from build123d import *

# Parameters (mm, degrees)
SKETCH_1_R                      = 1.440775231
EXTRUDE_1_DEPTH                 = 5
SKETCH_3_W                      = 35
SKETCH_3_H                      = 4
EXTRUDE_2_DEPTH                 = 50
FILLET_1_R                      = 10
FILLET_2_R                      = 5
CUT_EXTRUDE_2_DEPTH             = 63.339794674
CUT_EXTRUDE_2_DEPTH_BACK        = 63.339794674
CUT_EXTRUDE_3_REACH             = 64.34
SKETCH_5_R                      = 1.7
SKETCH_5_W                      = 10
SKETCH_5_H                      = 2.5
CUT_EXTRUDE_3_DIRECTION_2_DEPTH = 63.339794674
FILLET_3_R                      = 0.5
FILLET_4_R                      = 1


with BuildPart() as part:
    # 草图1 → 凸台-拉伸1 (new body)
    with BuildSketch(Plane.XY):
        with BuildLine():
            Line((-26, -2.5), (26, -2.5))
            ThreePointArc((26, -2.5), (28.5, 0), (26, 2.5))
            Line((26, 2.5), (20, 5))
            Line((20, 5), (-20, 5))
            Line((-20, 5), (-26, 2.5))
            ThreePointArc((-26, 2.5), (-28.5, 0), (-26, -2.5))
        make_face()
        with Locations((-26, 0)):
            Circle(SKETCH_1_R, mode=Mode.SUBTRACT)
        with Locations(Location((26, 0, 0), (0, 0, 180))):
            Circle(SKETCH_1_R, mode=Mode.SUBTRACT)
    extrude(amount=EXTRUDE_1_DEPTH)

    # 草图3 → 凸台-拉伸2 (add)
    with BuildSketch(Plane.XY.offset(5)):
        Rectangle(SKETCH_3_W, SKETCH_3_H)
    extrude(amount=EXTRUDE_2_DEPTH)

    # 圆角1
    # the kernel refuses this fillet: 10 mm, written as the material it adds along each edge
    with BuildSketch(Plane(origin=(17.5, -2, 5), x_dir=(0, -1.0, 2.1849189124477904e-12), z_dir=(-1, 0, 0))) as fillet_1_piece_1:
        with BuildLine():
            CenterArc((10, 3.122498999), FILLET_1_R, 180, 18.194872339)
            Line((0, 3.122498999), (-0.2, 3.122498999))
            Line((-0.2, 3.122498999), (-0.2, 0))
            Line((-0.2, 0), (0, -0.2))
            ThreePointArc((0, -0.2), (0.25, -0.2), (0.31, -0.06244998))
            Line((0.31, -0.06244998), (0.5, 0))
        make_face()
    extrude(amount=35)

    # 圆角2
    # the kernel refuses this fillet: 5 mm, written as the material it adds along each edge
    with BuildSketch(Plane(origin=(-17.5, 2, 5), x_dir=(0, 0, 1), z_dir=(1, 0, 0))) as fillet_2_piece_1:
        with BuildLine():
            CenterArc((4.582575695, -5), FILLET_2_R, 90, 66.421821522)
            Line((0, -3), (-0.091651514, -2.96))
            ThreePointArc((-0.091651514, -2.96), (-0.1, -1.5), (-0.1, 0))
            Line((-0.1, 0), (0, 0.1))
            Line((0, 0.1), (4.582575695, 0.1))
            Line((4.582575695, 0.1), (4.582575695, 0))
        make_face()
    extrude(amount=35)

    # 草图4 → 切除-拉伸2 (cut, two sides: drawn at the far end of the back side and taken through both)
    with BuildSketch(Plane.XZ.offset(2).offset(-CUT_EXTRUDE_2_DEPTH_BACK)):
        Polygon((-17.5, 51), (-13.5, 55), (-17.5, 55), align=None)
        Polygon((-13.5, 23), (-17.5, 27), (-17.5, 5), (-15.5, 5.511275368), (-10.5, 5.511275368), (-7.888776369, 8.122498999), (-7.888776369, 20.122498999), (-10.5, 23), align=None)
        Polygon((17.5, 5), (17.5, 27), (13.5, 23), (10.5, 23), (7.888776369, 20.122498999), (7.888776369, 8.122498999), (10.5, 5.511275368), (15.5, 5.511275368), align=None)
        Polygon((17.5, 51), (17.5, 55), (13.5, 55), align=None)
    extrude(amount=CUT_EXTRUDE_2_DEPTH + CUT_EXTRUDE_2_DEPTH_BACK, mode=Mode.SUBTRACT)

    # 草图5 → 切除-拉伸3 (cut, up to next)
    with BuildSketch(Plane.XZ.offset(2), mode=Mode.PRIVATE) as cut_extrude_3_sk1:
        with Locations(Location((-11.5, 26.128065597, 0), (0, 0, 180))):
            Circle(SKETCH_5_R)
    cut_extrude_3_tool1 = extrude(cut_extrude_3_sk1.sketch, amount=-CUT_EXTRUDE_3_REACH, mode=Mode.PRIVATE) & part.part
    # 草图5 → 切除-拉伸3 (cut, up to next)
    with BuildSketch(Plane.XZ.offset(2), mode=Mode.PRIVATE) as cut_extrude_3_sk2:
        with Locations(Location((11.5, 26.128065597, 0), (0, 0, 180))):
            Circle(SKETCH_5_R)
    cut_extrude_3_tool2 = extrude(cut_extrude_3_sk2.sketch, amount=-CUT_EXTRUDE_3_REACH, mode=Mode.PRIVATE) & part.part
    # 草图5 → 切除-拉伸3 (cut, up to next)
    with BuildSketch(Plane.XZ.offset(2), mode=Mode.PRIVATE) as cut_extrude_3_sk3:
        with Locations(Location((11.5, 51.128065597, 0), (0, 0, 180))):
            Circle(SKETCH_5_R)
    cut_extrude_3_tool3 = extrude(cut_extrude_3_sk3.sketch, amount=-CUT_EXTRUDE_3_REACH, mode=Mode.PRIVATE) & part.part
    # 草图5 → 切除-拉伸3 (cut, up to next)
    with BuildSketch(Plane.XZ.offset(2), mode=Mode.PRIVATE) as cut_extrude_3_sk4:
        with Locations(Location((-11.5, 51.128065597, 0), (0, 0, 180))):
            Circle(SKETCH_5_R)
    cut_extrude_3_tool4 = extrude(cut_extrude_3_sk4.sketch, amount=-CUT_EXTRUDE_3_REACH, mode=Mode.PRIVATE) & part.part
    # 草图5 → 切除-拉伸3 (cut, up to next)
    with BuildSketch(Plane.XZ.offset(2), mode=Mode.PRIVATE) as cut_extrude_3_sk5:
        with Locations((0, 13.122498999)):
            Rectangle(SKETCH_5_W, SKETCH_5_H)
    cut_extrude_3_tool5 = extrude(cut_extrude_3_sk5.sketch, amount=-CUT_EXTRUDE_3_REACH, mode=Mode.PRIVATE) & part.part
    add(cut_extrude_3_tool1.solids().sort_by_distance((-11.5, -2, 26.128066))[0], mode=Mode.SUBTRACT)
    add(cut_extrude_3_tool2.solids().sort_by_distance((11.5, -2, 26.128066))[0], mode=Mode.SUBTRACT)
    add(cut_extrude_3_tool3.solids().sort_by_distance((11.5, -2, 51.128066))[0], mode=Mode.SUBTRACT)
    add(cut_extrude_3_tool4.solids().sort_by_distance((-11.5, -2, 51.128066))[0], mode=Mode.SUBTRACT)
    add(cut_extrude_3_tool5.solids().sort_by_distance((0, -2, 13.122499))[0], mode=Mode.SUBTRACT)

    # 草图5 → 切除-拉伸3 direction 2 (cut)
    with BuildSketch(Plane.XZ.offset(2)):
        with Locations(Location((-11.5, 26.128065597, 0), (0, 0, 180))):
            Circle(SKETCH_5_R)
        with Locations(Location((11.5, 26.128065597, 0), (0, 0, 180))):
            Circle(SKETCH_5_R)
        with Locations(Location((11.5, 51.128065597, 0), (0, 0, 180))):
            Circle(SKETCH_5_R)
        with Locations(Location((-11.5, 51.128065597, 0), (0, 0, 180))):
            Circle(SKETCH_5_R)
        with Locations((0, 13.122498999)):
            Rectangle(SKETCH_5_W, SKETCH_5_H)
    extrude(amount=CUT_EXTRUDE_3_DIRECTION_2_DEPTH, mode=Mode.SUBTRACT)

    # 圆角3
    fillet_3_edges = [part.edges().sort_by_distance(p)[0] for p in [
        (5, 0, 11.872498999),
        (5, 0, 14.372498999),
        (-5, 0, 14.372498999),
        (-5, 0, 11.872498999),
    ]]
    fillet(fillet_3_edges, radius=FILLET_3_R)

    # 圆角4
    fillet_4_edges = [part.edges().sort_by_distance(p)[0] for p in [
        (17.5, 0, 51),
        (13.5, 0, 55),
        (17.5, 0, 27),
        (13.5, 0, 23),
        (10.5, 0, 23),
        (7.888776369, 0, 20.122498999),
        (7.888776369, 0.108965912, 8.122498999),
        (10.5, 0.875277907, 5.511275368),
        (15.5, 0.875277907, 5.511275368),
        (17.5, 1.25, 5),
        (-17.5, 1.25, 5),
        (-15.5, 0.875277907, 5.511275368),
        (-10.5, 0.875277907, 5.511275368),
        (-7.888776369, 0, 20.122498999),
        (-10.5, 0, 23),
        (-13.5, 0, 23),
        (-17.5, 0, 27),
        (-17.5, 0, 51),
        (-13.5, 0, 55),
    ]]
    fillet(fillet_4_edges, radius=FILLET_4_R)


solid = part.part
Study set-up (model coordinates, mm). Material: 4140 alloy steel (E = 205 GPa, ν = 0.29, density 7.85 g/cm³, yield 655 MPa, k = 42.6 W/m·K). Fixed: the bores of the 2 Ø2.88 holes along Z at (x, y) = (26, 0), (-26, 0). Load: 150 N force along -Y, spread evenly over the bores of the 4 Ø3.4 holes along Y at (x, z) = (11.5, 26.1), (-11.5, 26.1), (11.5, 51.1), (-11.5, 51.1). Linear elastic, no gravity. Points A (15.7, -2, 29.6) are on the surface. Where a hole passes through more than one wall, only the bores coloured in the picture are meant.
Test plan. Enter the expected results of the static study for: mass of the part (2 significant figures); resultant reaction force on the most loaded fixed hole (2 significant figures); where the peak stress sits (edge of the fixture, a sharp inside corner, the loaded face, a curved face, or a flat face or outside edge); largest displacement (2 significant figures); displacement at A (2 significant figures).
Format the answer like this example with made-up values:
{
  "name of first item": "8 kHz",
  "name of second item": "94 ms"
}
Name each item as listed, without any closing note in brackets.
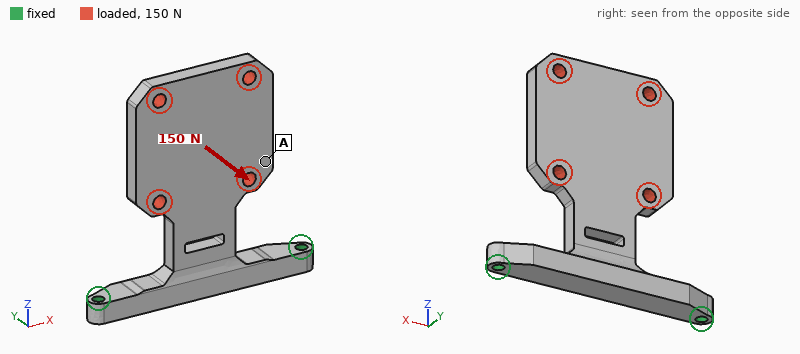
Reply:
{
  "mass of the part": "58 g",
  "resultant reaction force on the most loaded fixed hole": "110 N",
  "where the peak stress sits": "a curved face",
  "largest displacement": "0.45 mm",
  "displacement at A": "0.20 mm"
}
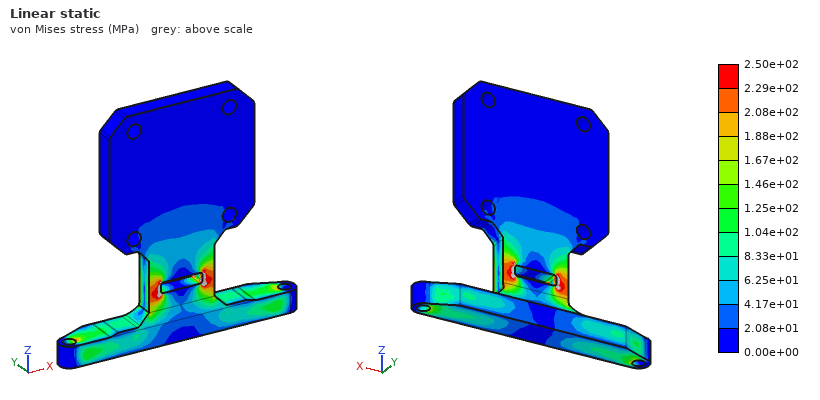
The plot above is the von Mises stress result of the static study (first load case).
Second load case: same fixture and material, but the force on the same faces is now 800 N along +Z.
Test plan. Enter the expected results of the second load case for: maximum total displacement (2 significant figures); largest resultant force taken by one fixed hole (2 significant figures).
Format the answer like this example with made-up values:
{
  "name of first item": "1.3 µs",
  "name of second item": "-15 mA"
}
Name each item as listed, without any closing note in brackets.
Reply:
{
  "maximum total displacement": "33 µm",
  "largest resultant force taken by one fixed hole": "480 N"
}
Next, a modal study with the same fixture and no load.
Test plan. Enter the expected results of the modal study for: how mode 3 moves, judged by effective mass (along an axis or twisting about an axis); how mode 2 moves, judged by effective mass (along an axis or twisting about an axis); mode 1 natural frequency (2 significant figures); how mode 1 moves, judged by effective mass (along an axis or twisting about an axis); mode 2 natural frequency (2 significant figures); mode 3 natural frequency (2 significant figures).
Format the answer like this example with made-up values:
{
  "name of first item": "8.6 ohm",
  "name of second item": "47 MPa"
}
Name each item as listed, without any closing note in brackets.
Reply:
{
  "how mode 3 moves, judged by effective mass": "twisting about Z",
  "how mode 2 moves, judged by effective mass": "along X",
  "mode 1 natural frequency": "590 Hz",
  "how mode 1 moves, judged by effective mass": "along Y",
  "mode 2 natural frequency": "2200 Hz",
  "mode 3 natural frequency": "2600 Hz"
}
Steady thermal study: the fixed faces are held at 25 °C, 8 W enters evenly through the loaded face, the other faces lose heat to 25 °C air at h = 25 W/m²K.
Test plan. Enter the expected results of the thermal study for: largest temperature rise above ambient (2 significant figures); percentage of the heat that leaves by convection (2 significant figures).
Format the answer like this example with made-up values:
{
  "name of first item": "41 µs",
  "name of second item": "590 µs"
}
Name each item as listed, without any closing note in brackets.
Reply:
{
  "largest temperature rise above ambient": "71 K",
  "percentage of the heat that leaves by convection": "63 %"
}
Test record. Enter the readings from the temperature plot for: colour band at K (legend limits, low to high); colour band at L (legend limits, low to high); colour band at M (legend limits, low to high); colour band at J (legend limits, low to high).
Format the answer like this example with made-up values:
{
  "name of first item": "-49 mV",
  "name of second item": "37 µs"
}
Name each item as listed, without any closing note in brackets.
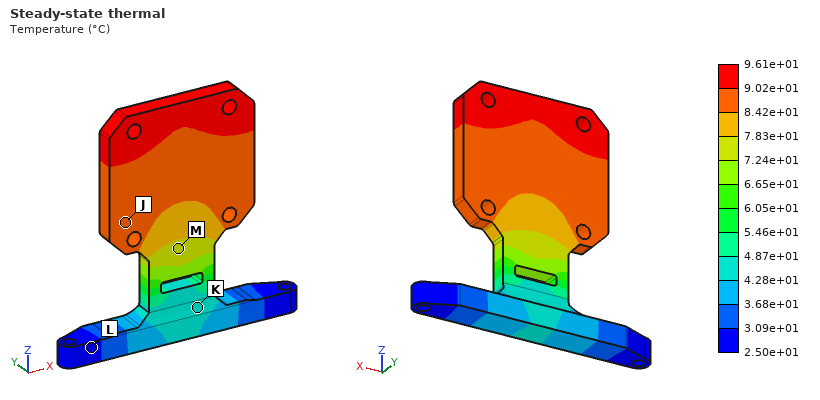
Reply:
{
  "colour band at K": "4.28e+01 to 4.87e+01 °C",
  "colour band at L": "2.50e+01 to 3.09e+01 °C",
  "colour band at M": "7.24e+01 to 7.83e+01 °C",
  "colour band at J": "8.42e+01 to 9.02e+01 °C"
}
